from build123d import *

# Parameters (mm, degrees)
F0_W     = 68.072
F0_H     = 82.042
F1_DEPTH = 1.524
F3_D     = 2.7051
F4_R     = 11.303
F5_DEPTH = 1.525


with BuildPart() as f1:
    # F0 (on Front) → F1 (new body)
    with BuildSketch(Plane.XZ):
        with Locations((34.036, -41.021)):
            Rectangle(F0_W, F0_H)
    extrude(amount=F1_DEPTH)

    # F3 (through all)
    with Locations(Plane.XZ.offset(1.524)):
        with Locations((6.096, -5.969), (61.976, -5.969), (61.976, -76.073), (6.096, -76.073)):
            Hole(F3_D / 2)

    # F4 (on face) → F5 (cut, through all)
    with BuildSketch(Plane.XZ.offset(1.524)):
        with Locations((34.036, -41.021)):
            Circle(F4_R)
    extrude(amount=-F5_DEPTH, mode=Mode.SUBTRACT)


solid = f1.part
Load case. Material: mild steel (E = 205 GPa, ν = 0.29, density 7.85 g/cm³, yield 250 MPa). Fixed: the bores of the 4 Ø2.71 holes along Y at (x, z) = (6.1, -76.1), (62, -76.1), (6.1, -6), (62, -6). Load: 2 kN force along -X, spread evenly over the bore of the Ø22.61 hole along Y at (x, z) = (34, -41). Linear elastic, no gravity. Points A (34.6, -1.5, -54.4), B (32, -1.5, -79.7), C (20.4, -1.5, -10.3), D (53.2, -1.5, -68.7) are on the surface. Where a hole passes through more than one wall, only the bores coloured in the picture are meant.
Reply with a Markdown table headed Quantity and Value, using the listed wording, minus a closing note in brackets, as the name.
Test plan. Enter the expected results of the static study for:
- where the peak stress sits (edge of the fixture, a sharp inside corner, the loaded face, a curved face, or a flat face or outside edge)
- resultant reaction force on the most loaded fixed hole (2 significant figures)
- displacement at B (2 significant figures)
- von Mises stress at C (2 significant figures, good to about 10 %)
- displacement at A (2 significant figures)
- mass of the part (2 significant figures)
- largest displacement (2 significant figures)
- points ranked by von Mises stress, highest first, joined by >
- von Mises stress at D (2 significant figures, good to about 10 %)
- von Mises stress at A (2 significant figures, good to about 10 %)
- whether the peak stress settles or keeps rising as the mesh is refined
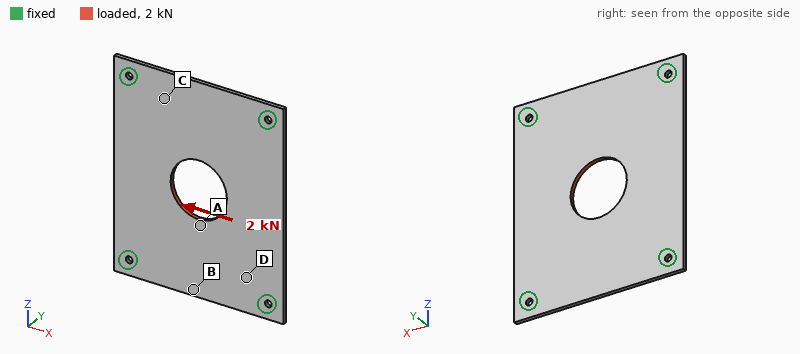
| Quantity | Value |
|---|---|
| where the peak stress sits | edge of the fixture |
| resultant reaction force on the most loaded fixed hole | 580 N |
| displacement at B | 1.6 µm |
| von Mises stress at C | 18 MPa |
| displacement at A | 4.7 µm |
| mass of the part | 62 g |
| largest displacement | 6.2 µm |
| points ranked by von Mises stress, highest first, joined by > | A > D > C > B |
| von Mises stress at D | 23 MPa |
| von Mises stress at A | 31 MPa |
| whether the peak stress settles or keeps rising as the mesh is refined | keeps rising |
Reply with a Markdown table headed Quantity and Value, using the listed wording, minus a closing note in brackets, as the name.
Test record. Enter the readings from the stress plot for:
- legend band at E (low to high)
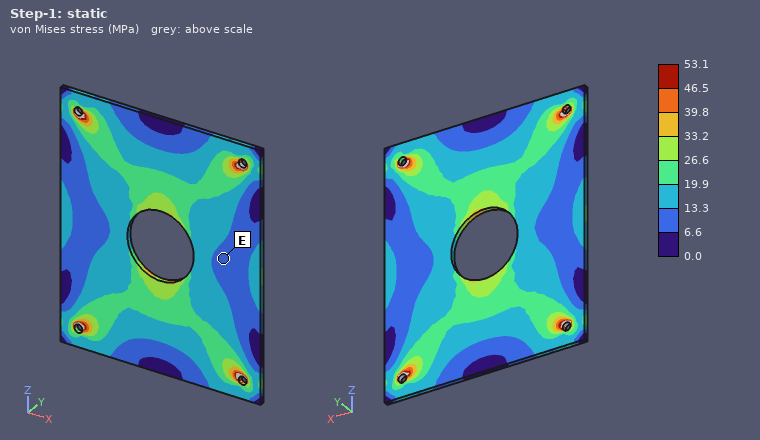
| Quantity | Value |
|---|---|
| legend band at E | 6.6 to 13.3 MPa |
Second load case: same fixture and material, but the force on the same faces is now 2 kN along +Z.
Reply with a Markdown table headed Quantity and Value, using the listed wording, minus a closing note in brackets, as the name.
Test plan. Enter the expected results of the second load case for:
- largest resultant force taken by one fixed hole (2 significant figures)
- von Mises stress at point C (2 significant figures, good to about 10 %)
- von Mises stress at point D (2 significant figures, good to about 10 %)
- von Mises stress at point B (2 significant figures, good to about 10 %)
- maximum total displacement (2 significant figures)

| Quantity | Value |
|---|---|
| largest resultant force taken by one fixed hole | 540 N |
| von Mises stress at point C | 12 MPa |
| von Mises stress at point D | 20 MPa |
| von Mises stress at point B | 10 MPa |
| maximum total displacement | 4.5 µm |
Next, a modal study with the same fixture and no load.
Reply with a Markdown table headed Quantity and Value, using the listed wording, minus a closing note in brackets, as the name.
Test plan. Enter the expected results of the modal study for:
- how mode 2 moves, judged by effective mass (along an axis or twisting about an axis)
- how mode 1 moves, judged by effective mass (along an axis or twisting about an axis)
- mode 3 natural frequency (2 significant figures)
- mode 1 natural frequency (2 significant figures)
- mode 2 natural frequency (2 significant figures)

| Quantity | Value |
|---|---|
| how mode 2 moves, judged by effective mass | twisting about Z |
| how mode 1 moves, judged by effective mass | along Y |
| mode 3 natural frequency | 2400 Hz |
| mode 1 natural frequency | 1300 Hz |
| mode 2 natural frequency | 1900 Hz |
